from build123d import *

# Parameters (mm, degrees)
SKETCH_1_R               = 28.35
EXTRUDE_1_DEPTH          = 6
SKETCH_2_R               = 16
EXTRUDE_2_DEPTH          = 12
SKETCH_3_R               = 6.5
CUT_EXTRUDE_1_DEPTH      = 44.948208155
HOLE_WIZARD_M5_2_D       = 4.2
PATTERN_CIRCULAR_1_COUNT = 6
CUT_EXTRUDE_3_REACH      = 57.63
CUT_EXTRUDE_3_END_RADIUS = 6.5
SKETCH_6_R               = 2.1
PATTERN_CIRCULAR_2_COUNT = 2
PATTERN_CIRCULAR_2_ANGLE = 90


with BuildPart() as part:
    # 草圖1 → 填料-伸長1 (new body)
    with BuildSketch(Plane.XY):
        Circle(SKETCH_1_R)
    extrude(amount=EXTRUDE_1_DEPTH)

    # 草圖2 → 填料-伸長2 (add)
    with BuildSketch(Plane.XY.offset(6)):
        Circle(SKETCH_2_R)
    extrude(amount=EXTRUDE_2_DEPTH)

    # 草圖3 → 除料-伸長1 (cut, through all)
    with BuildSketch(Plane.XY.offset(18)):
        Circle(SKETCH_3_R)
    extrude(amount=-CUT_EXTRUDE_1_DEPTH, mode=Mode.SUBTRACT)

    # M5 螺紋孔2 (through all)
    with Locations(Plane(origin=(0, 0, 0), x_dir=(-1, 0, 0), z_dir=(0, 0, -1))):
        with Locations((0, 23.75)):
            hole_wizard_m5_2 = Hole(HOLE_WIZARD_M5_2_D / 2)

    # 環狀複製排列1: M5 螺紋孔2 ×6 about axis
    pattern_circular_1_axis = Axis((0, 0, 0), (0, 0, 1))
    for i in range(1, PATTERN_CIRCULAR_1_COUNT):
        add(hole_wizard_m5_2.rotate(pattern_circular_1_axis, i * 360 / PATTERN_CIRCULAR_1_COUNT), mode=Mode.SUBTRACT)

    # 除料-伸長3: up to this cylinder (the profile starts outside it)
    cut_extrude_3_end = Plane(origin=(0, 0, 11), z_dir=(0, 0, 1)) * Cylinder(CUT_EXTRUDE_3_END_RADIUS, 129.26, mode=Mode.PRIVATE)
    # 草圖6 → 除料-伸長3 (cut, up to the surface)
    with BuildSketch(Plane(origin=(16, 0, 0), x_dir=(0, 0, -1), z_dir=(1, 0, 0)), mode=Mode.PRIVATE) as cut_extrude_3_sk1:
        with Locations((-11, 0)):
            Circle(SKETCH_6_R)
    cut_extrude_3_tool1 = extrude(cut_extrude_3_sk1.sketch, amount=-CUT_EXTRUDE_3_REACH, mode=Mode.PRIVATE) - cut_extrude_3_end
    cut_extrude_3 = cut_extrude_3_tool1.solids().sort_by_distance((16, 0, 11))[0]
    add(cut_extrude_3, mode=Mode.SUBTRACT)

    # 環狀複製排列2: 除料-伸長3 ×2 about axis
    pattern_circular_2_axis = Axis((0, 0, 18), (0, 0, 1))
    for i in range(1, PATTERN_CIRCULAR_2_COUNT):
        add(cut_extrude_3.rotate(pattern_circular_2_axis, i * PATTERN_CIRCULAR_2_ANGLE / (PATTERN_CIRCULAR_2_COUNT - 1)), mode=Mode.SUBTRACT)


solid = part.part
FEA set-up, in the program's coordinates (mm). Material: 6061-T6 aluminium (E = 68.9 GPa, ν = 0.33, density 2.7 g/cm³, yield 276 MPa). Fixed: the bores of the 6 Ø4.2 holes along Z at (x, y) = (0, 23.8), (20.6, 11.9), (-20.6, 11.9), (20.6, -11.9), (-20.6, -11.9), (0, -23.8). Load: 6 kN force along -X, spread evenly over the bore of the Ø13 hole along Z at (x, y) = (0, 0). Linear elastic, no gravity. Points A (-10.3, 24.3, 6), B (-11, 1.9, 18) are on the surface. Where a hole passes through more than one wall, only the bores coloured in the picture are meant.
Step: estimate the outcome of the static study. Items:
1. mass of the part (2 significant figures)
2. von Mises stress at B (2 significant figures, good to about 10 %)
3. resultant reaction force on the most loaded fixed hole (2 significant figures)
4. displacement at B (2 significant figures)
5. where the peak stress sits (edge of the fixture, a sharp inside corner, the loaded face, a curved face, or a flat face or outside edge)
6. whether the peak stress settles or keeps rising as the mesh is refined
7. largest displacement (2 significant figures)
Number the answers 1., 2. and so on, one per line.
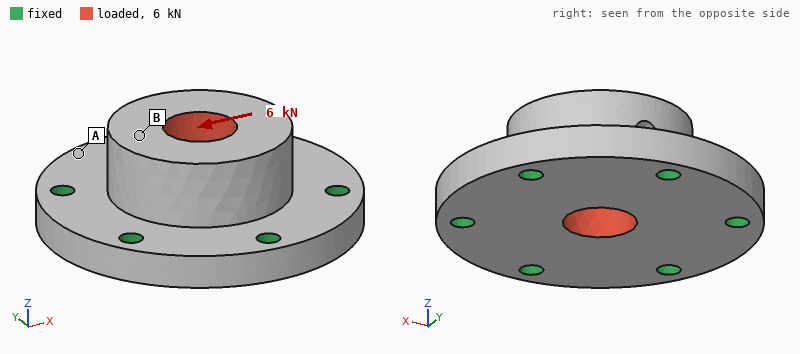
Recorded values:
1. 58 g
2. 9.7 MPa
3. 1.4 kN
4. 9.3 µm
5. edge of the fixture
6. keeps rising
7. 9.8 µm
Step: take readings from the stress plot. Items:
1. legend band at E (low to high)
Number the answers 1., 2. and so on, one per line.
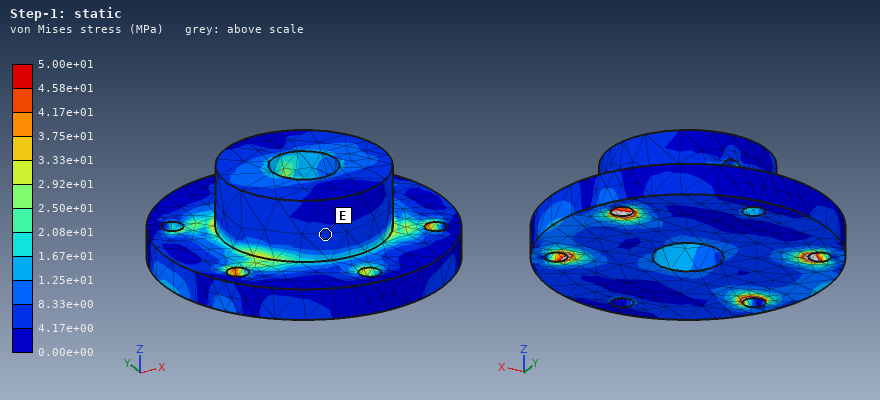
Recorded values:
1. 4.17e+00 to 8.33e+00 MPa
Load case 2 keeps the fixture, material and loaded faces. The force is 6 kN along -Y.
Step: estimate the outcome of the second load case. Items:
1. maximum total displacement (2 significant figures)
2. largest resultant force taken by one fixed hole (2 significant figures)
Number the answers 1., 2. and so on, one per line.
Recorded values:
1. 9.8 µm
2. 1.6 kN
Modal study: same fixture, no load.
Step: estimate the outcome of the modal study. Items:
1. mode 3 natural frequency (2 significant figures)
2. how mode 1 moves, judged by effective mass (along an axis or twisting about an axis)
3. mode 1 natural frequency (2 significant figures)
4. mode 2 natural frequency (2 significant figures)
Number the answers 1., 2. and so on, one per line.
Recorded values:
1. 24 kHz
2. along Z
3. 20 kHz
4. 24 kHz
